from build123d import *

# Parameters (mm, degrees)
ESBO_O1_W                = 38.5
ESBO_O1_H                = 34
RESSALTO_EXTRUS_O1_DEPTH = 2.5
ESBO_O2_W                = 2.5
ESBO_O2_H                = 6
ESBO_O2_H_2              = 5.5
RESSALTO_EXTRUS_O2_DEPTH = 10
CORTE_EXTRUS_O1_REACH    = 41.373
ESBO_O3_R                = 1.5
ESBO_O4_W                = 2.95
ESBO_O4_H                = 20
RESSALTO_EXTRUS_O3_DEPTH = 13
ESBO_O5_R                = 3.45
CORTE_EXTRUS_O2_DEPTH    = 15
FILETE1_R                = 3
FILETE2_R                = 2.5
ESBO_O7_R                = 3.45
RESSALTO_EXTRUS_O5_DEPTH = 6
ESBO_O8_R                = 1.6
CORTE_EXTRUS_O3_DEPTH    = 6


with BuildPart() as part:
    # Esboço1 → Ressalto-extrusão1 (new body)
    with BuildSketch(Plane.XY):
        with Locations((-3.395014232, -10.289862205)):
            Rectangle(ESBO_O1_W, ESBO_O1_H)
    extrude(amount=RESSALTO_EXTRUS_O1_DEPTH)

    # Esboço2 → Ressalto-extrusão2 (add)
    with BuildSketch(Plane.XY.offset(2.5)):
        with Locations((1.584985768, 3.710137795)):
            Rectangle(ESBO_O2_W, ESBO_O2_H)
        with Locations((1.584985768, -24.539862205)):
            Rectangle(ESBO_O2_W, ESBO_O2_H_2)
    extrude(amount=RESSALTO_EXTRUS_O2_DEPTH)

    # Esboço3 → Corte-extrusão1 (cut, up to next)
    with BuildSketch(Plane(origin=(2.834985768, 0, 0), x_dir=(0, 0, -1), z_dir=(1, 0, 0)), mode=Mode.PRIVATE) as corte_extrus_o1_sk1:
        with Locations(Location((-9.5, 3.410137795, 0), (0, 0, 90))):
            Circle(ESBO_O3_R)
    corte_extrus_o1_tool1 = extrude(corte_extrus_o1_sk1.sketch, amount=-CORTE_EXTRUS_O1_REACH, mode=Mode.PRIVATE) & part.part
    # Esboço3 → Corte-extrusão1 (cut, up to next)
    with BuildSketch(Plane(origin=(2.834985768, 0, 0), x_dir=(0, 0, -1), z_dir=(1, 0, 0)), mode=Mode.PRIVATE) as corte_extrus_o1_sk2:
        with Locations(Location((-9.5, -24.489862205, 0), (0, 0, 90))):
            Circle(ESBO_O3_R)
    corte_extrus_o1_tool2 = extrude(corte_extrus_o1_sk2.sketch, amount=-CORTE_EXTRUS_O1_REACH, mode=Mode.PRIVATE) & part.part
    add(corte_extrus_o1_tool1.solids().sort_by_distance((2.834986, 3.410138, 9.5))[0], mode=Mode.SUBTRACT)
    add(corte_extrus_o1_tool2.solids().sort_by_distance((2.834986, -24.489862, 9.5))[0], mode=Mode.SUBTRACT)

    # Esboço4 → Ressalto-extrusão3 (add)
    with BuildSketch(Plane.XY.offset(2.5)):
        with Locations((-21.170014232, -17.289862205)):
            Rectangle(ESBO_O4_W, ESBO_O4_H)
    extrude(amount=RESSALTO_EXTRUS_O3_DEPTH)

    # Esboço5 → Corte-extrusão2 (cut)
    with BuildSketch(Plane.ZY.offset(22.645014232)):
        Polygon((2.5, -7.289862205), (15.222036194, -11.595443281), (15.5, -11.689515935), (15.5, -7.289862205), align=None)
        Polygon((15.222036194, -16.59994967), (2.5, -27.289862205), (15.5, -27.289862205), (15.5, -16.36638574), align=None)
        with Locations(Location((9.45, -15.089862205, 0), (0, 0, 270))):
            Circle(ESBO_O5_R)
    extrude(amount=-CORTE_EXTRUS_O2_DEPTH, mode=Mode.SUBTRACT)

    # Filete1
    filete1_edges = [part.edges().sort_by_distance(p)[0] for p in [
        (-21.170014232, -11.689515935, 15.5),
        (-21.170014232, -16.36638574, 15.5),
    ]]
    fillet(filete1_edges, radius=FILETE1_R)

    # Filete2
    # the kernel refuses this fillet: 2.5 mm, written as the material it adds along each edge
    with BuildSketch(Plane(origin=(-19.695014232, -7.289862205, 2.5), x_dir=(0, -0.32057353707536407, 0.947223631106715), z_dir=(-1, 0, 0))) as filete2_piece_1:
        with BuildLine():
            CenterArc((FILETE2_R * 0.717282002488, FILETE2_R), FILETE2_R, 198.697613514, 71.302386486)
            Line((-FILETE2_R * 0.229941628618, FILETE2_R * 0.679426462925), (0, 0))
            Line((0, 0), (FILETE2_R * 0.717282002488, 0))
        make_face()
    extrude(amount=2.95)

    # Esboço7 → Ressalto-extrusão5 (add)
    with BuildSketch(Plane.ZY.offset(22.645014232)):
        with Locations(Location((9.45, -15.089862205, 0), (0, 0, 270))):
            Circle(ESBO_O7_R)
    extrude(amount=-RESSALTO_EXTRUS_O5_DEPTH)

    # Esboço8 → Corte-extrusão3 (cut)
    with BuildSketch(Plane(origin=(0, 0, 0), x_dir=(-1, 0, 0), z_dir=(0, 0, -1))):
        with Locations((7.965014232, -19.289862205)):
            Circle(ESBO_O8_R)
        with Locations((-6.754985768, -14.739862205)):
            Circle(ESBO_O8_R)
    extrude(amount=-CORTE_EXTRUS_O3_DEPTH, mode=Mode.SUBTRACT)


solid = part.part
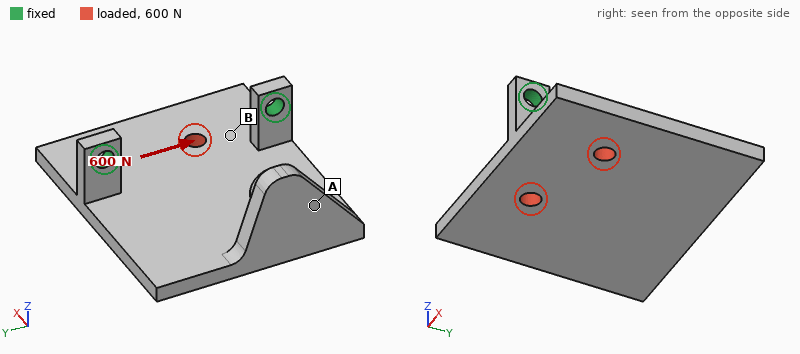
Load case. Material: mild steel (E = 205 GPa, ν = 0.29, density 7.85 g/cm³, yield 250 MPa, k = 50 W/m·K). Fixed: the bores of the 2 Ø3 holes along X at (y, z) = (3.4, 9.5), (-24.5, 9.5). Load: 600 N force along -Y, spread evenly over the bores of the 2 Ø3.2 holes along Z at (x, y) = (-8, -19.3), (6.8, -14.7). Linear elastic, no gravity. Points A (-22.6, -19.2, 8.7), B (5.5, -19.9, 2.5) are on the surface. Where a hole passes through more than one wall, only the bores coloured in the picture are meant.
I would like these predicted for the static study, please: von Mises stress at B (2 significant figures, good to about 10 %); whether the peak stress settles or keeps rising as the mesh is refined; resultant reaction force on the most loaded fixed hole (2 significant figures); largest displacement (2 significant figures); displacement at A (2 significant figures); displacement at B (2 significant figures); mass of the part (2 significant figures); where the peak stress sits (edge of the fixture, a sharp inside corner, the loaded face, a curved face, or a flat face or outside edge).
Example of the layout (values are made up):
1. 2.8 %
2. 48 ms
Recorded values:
1. 25 MPa
2. keeps rising
3. 320 N
4. 12 µm
5. 11 µm
6. 5.8 µm
7. 32 g
8. edge of the fixture
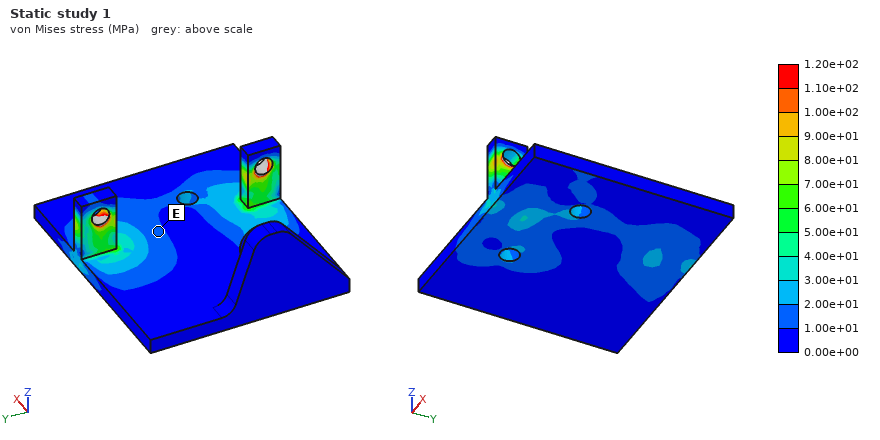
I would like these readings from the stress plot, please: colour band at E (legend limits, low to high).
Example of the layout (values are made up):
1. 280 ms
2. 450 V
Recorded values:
1. 1.00e+01 to 2.00e+01 MPa
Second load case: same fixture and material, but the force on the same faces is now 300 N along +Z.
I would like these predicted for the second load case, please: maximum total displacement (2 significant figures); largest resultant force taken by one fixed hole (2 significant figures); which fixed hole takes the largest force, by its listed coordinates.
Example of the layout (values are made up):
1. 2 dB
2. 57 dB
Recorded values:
1. 62 µm
2. 240 N
3. (-24.5, 9.5)
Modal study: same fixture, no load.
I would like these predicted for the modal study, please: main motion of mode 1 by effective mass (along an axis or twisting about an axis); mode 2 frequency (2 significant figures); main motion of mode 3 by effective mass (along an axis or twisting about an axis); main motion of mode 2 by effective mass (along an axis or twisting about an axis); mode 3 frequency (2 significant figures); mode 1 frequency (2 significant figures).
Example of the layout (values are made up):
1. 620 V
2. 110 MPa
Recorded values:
1. along Z
2. 3700 Hz
3. along X
4. along Y
5. 4700 Hz
6. 1200 Hz
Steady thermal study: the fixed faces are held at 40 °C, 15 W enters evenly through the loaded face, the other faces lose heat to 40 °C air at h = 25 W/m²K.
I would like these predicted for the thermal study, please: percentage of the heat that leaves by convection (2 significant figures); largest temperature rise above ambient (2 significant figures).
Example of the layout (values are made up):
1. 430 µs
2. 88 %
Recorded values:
1. 34 %
2. 82 K
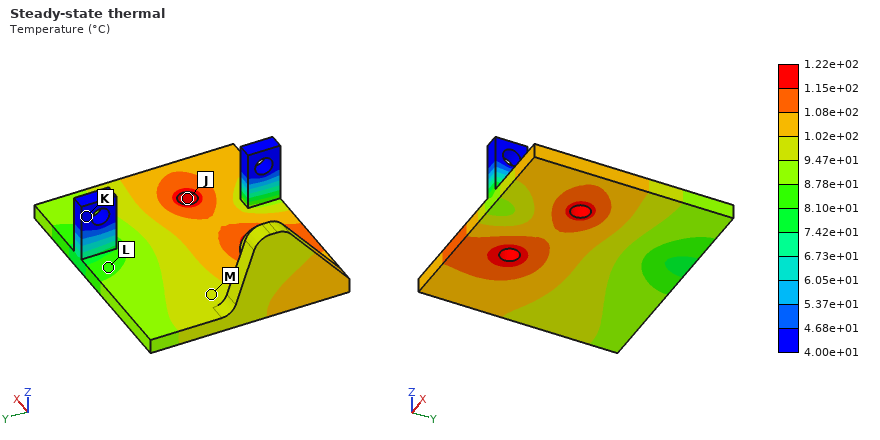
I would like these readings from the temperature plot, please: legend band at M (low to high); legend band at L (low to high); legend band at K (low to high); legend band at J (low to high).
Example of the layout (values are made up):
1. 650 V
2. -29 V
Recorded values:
1. 9.47e+01 to 1.02e+02 °C
2. 8.10e+01 to 8.78e+01 °C
3. 4.00e+01 to 4.68e+01 °C
4. 1.15e+02 to 1.22e+02 °C
